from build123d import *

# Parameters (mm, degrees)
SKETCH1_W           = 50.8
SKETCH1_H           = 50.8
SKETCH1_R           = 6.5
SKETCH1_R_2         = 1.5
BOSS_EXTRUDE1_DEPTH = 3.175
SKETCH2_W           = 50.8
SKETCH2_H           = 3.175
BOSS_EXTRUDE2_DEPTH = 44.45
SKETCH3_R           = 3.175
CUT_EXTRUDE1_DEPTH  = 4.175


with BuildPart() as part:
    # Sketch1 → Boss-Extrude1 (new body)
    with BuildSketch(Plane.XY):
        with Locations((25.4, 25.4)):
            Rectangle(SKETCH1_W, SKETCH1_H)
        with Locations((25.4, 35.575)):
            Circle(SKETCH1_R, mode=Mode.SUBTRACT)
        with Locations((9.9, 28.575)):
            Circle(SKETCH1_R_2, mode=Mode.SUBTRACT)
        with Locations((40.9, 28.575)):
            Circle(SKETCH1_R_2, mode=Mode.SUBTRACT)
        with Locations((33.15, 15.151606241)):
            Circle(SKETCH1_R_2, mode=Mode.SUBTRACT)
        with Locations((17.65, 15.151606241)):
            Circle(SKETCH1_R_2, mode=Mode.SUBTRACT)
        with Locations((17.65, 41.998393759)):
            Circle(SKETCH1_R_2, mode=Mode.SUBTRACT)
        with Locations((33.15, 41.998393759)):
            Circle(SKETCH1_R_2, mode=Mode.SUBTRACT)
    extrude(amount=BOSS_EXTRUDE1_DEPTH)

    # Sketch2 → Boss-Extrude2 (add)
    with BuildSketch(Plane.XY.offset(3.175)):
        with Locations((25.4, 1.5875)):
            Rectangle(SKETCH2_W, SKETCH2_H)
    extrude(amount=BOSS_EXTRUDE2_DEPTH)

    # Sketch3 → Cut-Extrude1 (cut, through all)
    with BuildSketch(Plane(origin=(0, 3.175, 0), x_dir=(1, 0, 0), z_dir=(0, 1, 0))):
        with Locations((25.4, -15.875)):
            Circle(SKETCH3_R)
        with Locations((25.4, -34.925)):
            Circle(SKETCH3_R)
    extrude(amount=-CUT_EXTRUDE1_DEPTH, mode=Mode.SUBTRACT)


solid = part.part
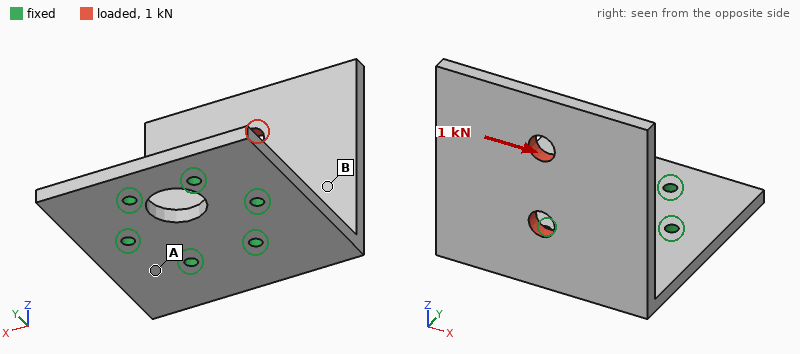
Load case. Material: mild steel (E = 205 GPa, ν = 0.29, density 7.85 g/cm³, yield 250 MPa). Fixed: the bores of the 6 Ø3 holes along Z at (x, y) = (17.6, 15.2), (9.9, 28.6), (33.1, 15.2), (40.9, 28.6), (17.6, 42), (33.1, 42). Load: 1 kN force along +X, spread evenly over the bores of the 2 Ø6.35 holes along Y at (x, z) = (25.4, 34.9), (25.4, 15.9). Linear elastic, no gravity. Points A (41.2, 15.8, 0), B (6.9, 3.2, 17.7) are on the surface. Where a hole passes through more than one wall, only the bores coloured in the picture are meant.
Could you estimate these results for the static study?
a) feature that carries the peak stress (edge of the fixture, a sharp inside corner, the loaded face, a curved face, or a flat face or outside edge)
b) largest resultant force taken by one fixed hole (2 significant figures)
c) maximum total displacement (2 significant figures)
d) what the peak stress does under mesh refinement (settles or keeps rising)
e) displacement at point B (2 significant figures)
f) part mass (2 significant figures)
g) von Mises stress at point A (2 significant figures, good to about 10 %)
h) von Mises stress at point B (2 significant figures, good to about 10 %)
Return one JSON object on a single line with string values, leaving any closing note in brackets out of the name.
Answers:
{"feature that carries the peak stress": "edge of the fixture", "largest resultant force taken by one fixed hole": "1.2 kN", "maximum total displacement": "0.19 mm", "what the peak stress does under mesh refinement": "keeps rising", "displacement at point B": "0.088 mm", "part mass": "110 g", "von Mises stress at point A": "110 MPa", "von Mises stress at point B": "40 MPa"}
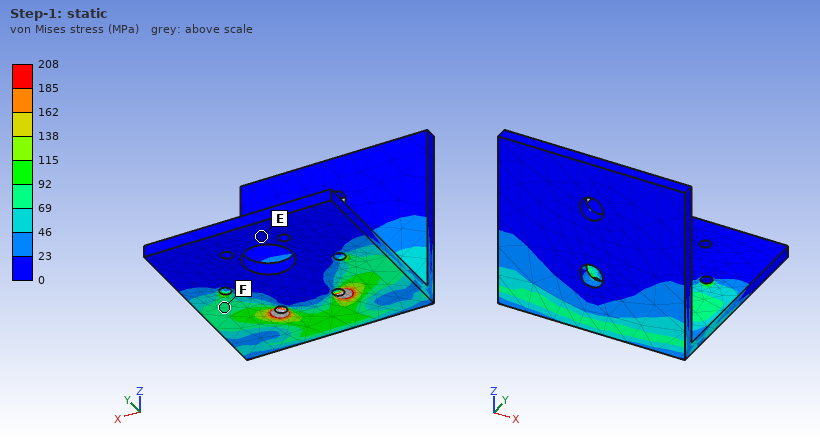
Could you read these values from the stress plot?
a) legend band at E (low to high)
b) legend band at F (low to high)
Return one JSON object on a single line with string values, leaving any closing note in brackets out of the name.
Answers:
{"legend band at E": "0 to 23 MPa", "legend band at F": "69 to 92 MPa"}
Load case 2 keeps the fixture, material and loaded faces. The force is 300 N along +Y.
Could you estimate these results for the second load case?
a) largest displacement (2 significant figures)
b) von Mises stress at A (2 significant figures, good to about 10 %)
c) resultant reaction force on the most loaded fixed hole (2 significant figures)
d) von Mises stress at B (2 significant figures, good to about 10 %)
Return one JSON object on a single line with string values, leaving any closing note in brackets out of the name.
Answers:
{"largest displacement": "0.28 mm", "von Mises stress at A": "42 MPa", "resultant reaction force on the most loaded fixed hole": "170 N", "von Mises stress at B": "35 MPa"}
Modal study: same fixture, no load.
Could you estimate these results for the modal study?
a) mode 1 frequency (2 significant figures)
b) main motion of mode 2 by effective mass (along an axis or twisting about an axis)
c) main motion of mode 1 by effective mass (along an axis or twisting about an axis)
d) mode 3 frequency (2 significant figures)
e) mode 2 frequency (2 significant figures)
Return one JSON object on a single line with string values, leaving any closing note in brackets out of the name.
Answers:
{"mode 1 frequency": "850 Hz", "main motion of mode 2 by effective mass": "along X", "main motion of mode 1 by effective mass": "along Y", "mode 3 frequency": "2700 Hz", "mode 2 frequency": "1700 Hz"}
